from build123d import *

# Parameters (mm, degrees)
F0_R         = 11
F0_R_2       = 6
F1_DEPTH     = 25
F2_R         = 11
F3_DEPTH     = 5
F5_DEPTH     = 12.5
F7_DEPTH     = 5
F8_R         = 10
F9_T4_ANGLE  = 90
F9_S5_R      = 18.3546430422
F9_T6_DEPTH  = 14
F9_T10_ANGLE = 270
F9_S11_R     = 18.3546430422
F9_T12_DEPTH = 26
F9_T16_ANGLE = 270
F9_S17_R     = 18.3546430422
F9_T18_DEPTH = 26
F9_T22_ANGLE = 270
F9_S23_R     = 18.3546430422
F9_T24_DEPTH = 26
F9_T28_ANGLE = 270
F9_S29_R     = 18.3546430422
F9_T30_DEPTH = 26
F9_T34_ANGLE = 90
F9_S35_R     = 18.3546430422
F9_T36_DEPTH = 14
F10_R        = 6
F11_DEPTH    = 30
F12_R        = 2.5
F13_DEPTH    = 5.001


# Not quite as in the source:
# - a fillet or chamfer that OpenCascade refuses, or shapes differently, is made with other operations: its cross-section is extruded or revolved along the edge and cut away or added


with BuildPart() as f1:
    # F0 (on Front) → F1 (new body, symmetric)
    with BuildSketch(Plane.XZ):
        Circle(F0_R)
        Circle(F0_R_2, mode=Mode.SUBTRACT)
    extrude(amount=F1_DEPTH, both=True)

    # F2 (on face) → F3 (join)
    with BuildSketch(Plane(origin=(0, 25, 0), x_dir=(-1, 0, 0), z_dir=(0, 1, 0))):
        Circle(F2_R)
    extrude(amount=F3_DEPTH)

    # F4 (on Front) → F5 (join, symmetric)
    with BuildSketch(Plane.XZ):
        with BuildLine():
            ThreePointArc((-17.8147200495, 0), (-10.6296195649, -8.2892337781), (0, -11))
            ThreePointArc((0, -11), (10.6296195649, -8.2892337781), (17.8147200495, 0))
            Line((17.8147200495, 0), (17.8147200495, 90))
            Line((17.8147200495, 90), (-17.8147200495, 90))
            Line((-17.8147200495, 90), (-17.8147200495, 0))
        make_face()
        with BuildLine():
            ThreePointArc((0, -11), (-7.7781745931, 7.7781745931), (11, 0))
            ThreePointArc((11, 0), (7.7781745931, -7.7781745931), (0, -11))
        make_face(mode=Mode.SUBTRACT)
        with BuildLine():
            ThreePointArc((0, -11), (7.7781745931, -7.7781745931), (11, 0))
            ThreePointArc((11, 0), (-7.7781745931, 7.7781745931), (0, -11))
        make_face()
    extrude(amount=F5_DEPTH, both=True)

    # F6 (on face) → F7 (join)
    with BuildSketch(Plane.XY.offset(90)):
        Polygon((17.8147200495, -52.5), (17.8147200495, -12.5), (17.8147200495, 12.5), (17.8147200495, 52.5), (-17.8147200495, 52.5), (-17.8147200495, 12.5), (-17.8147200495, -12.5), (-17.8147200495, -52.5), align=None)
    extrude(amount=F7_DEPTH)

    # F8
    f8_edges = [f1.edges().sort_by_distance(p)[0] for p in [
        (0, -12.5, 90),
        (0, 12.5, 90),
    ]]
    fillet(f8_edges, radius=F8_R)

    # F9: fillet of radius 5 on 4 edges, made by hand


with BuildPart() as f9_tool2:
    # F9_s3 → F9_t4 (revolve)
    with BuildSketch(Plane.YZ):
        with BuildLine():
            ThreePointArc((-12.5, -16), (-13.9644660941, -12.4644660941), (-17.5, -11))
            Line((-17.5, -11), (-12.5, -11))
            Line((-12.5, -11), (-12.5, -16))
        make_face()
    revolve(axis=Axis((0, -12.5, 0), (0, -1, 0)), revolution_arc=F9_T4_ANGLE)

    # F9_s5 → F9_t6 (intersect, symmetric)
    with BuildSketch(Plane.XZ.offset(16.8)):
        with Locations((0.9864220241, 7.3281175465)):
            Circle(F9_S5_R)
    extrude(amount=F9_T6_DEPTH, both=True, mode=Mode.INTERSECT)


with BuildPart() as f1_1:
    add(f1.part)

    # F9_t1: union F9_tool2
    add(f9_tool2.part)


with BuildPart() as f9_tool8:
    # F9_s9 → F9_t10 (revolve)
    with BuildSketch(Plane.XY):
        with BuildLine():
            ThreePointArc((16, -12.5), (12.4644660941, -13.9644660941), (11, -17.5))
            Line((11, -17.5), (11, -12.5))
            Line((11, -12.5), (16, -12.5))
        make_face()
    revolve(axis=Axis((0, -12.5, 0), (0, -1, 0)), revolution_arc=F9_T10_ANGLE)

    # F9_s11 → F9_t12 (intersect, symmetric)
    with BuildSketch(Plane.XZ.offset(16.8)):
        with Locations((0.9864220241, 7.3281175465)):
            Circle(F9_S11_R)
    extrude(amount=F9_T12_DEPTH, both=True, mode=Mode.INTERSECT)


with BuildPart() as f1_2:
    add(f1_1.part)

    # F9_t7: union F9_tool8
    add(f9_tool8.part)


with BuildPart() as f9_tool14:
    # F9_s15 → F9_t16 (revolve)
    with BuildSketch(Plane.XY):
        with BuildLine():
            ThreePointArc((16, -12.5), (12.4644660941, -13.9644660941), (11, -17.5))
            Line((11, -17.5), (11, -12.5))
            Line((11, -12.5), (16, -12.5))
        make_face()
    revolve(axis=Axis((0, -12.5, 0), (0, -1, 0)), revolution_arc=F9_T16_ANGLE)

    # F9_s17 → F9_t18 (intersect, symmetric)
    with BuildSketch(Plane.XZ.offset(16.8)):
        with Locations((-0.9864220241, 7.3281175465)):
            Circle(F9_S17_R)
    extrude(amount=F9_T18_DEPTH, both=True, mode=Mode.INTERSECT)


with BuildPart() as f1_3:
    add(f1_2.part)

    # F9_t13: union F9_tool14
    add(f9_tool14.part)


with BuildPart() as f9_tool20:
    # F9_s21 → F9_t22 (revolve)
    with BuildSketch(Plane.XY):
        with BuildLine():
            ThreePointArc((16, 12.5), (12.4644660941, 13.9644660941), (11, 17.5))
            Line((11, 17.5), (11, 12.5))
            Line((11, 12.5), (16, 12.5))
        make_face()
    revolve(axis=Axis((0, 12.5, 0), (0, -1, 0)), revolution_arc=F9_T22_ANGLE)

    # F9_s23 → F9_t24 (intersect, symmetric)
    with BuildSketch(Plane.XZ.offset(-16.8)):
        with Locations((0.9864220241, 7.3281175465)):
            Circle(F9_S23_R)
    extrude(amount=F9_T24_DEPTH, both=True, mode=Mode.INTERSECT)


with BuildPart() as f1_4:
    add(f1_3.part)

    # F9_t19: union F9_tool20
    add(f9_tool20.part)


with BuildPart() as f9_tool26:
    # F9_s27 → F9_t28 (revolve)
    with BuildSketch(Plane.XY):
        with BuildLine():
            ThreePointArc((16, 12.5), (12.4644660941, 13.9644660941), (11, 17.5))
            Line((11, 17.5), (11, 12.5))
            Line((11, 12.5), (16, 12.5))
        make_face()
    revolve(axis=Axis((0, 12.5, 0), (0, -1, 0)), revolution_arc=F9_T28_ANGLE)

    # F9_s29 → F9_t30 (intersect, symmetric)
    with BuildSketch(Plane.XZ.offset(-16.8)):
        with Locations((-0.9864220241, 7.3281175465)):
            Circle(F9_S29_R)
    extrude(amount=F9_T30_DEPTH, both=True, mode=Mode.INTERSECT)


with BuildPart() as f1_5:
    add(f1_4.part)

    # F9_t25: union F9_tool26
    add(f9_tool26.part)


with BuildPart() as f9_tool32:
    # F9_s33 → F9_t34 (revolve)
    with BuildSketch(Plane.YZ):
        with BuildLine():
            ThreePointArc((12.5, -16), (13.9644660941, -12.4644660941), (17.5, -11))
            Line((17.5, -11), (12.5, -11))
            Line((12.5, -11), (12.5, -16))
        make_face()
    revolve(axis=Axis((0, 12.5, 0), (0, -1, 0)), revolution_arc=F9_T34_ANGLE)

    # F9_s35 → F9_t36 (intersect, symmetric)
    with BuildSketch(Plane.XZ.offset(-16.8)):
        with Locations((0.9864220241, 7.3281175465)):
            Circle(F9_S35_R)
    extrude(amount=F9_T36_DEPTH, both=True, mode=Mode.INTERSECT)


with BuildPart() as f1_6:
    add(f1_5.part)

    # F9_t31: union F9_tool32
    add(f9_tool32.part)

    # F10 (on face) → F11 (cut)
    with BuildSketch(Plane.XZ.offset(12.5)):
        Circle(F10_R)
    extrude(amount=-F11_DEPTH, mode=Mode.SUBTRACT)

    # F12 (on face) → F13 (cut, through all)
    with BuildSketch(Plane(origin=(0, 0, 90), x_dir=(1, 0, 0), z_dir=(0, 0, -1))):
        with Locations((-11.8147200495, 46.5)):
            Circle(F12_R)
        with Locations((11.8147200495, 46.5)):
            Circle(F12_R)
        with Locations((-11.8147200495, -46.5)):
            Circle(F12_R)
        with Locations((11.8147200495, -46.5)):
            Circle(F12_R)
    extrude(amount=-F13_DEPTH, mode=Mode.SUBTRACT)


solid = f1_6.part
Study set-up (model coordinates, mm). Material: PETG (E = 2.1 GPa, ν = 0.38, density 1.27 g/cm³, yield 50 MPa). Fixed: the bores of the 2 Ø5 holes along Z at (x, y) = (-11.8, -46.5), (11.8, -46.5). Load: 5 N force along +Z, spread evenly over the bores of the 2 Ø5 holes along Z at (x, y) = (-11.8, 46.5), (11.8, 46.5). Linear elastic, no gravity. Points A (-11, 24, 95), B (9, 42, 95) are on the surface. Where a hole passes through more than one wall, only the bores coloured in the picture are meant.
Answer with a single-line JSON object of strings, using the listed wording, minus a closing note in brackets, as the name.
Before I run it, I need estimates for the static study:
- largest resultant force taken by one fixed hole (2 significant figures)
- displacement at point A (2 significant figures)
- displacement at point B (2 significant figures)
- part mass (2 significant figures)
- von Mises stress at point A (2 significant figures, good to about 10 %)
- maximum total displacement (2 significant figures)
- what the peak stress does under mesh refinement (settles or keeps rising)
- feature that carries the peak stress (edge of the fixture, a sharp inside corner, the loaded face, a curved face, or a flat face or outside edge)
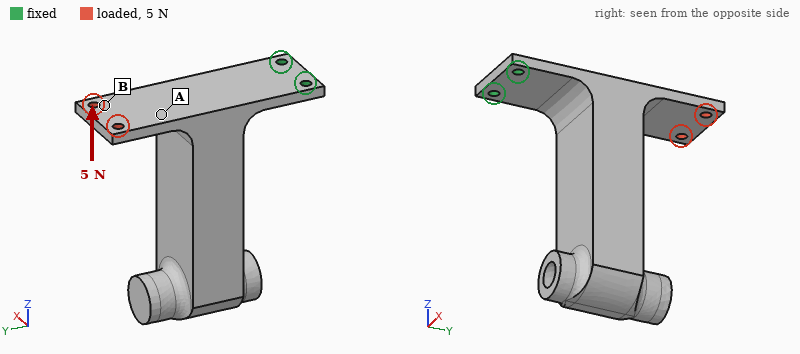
{"largest resultant force taken by one fixed hole": "2.5 N", "displacement at point A": "0.80 mm", "displacement at point B": "1.1 mm", "part mass": "140 g", "von Mises stress at point A": "0.68 MPa", "maximum total displacement": "1.7 mm", "what the peak stress does under mesh refinement": "keeps rising", "feature that carries the peak stress": "edge of the fixture"}
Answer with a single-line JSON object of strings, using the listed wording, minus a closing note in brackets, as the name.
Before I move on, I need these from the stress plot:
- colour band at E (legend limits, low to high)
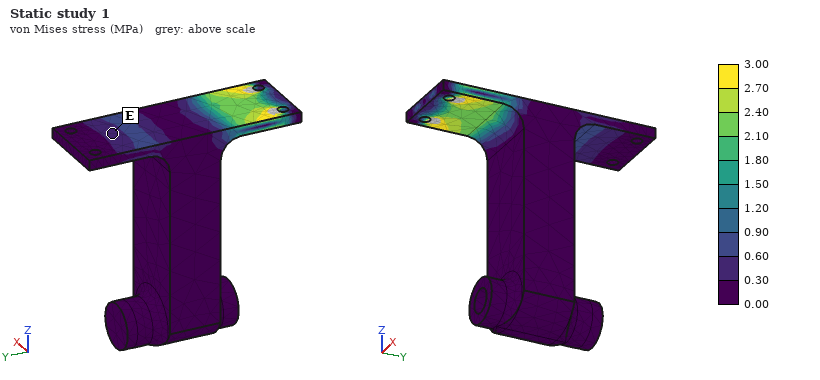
{"colour band at E": "0.30 to 0.60 MPa"}
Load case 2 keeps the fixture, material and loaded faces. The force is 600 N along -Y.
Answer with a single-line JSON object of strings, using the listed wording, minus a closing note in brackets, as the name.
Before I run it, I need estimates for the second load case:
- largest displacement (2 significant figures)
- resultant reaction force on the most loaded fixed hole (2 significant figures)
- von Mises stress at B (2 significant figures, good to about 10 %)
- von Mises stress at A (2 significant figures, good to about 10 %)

{"largest displacement": "0.41 mm", "resultant reaction force on the most loaded fixed hole": "300 N", "von Mises stress at B": "4.7 MPa", "von Mises stress at A": "3.5 MPa"}
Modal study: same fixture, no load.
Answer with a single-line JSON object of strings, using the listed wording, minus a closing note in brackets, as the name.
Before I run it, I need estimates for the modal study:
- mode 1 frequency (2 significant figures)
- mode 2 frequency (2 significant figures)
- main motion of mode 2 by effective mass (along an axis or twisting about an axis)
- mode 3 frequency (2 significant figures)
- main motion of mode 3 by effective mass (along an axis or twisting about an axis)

{"mode 1 frequency": "33 Hz", "mode 2 frequency": "62 Hz", "main motion of mode 2 by effective mass": "along X", "mode 3 frequency": "270 Hz", "main motion of mode 3 by effective mass": "along Z"}
